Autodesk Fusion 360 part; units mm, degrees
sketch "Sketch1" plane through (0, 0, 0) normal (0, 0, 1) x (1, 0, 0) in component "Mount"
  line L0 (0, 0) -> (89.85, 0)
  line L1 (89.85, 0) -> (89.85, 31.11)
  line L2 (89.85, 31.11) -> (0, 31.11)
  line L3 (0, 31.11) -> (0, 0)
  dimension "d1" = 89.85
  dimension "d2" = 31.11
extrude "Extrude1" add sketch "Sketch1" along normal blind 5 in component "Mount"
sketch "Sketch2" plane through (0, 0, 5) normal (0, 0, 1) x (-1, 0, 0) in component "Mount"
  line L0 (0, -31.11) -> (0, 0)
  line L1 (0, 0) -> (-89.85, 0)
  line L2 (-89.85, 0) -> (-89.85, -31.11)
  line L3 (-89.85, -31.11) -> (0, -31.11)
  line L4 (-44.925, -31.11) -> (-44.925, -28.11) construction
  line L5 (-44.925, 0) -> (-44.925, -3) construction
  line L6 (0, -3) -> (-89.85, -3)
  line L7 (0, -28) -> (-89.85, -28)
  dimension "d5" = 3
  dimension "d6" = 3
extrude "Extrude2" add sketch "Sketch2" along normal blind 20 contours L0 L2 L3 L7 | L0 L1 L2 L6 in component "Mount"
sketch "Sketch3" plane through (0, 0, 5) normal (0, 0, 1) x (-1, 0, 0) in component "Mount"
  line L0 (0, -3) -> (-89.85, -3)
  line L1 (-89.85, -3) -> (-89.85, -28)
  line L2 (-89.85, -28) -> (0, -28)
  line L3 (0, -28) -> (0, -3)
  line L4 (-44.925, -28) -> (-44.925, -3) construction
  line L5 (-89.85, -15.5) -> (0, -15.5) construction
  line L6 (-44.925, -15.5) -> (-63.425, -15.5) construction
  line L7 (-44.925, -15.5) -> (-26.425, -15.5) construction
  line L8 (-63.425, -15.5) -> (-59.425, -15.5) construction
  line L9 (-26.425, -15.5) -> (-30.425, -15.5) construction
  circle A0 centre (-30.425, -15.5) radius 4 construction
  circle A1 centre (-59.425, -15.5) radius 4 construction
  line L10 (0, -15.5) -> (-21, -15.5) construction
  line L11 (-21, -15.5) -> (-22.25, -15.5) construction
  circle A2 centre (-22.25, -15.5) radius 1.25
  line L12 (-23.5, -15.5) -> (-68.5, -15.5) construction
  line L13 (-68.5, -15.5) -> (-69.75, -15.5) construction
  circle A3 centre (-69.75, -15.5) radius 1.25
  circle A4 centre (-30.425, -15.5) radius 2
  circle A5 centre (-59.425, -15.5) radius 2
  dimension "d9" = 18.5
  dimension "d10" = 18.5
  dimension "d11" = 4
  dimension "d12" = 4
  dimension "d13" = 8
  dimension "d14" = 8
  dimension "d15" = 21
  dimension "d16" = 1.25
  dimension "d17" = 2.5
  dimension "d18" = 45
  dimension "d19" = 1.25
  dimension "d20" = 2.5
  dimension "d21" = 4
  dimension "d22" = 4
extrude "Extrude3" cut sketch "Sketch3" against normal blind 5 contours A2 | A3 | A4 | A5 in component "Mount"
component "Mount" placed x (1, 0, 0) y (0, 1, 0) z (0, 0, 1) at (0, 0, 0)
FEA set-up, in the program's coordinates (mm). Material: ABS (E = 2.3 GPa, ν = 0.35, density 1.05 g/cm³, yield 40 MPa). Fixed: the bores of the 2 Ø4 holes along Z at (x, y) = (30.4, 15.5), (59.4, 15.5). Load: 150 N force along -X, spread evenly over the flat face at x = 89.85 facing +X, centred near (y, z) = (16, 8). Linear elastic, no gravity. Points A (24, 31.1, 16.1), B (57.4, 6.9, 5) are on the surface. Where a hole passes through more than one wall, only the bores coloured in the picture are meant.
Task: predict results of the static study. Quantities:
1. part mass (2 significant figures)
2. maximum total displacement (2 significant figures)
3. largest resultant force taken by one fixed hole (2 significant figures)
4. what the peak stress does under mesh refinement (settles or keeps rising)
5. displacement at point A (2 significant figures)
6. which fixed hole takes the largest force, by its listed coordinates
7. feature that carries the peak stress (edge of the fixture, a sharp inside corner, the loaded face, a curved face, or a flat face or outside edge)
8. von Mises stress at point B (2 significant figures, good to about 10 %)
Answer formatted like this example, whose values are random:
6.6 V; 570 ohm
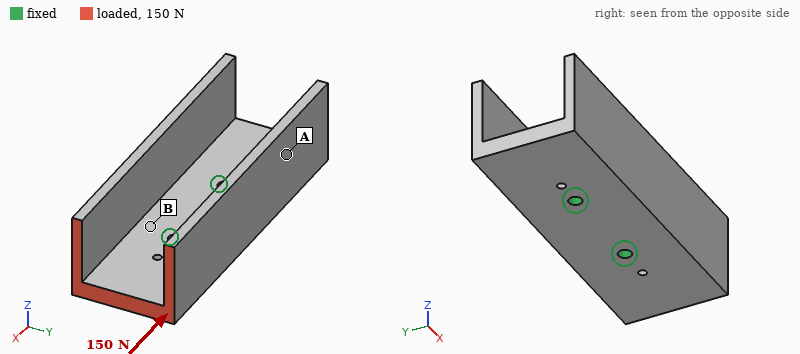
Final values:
26 g; 52 µm; 100 N; keeps rising; 22 µm; (59.4, 15.5); edge of the fixture; 0.79 MPa
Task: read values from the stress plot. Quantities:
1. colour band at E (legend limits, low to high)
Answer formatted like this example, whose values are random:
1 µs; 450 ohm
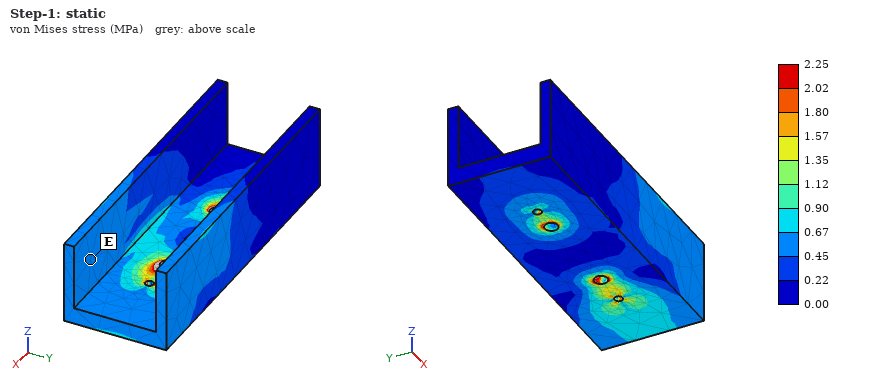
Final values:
0.45 to 0.67 MPa
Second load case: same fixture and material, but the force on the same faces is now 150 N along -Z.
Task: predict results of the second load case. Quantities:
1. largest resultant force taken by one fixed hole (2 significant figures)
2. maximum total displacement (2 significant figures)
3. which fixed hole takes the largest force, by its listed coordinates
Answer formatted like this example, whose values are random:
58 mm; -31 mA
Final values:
270 N; 0.43 mm; (59.4, 15.5)
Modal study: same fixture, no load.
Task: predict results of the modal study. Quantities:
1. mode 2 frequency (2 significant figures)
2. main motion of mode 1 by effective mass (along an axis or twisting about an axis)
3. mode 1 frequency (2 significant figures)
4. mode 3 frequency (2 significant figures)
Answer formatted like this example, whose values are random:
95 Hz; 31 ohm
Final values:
1000 Hz; along Y; 960 Hz; 1200 Hz
